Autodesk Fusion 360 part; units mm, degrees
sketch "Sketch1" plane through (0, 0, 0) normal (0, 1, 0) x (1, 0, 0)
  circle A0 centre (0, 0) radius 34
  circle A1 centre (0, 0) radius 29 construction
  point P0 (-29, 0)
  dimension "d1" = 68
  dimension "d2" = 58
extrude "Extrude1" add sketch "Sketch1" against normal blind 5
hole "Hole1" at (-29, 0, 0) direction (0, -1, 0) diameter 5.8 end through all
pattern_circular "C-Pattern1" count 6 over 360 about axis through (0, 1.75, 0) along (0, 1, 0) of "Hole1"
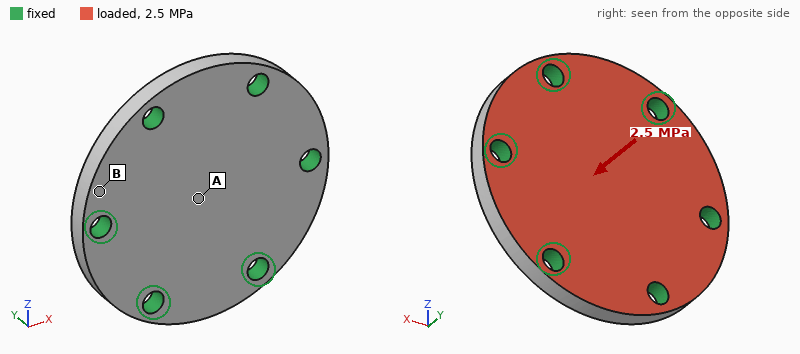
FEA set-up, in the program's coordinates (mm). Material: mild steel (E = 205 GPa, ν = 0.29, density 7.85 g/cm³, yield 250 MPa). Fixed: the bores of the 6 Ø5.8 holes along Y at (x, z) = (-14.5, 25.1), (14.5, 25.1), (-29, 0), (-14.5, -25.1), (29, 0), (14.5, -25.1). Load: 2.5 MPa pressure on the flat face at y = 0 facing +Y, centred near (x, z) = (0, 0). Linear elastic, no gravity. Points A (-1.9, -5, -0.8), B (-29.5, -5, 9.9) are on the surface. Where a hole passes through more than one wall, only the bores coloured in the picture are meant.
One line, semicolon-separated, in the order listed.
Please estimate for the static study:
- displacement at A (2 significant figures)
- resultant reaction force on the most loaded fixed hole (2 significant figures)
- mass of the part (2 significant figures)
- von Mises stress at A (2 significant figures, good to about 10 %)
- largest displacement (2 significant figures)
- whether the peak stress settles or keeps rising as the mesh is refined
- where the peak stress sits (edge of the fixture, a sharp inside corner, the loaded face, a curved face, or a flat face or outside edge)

14 µm; 1.4 kN; 140 g; 40 MPa; 14 µm; keeps rising; edge of the fixture
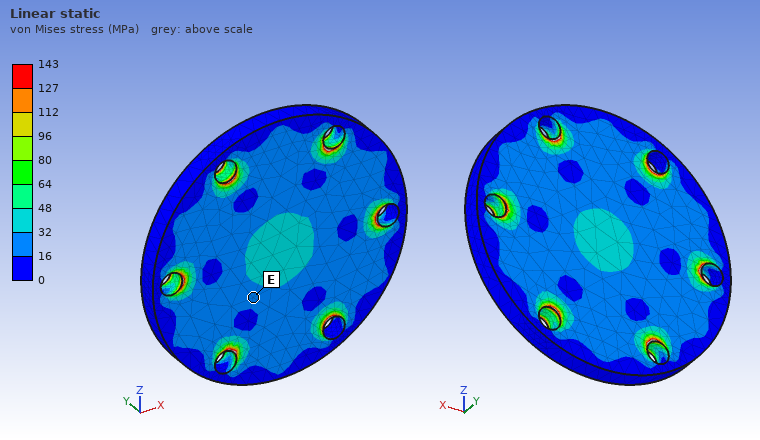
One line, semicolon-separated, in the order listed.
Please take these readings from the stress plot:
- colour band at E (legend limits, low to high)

16 to 32 MPa
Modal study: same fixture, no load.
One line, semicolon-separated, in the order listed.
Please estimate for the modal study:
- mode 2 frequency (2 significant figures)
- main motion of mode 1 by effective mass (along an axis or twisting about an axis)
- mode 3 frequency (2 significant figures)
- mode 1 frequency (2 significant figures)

25 kHz; along Y; 25 kHz; 13 kHz
